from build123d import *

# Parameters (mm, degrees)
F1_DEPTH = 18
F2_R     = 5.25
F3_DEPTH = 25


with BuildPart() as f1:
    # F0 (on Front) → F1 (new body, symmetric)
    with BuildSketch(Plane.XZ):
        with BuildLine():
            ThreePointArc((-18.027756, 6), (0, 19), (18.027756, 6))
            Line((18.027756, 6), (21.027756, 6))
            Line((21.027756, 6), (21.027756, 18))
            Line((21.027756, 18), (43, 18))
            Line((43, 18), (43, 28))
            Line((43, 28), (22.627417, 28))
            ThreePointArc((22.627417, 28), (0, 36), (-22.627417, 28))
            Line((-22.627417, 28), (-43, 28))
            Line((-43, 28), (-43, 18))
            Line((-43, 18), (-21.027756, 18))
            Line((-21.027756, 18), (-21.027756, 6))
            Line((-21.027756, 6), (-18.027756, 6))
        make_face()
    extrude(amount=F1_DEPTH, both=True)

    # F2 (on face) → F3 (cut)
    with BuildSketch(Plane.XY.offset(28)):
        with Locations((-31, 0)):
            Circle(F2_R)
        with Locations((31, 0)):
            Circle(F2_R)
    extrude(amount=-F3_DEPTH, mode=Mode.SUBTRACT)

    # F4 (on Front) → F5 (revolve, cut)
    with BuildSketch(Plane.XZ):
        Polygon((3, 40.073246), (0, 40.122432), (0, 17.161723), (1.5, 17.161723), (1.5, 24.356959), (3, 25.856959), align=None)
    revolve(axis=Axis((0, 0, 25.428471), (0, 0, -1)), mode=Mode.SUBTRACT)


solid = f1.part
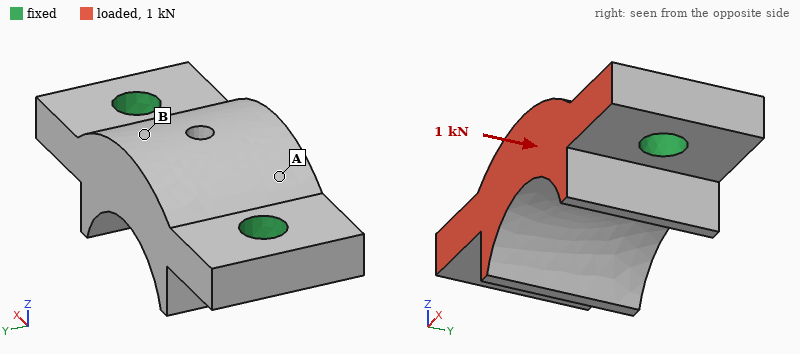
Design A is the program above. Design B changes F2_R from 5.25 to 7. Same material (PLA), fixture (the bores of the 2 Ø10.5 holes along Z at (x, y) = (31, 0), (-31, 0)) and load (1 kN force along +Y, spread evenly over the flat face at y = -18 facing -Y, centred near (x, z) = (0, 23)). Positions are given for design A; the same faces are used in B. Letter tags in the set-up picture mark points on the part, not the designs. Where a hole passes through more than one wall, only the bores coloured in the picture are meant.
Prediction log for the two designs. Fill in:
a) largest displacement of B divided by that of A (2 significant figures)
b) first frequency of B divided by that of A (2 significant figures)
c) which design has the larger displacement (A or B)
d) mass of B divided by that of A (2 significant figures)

0.82
1.2
A
0.97
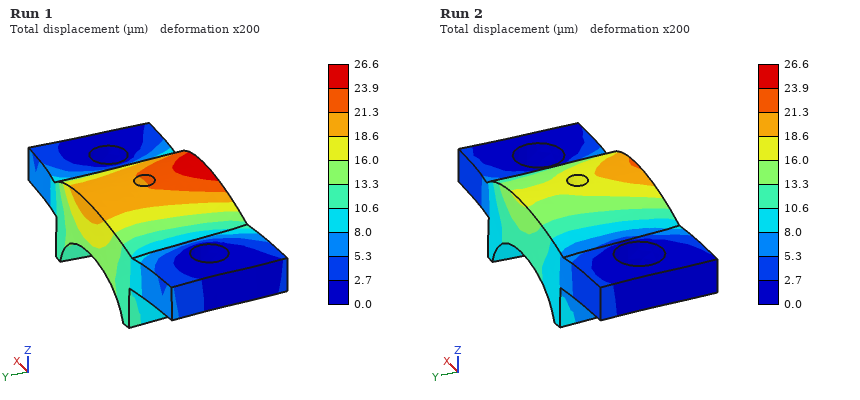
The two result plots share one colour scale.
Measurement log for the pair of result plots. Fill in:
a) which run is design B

Run 2
